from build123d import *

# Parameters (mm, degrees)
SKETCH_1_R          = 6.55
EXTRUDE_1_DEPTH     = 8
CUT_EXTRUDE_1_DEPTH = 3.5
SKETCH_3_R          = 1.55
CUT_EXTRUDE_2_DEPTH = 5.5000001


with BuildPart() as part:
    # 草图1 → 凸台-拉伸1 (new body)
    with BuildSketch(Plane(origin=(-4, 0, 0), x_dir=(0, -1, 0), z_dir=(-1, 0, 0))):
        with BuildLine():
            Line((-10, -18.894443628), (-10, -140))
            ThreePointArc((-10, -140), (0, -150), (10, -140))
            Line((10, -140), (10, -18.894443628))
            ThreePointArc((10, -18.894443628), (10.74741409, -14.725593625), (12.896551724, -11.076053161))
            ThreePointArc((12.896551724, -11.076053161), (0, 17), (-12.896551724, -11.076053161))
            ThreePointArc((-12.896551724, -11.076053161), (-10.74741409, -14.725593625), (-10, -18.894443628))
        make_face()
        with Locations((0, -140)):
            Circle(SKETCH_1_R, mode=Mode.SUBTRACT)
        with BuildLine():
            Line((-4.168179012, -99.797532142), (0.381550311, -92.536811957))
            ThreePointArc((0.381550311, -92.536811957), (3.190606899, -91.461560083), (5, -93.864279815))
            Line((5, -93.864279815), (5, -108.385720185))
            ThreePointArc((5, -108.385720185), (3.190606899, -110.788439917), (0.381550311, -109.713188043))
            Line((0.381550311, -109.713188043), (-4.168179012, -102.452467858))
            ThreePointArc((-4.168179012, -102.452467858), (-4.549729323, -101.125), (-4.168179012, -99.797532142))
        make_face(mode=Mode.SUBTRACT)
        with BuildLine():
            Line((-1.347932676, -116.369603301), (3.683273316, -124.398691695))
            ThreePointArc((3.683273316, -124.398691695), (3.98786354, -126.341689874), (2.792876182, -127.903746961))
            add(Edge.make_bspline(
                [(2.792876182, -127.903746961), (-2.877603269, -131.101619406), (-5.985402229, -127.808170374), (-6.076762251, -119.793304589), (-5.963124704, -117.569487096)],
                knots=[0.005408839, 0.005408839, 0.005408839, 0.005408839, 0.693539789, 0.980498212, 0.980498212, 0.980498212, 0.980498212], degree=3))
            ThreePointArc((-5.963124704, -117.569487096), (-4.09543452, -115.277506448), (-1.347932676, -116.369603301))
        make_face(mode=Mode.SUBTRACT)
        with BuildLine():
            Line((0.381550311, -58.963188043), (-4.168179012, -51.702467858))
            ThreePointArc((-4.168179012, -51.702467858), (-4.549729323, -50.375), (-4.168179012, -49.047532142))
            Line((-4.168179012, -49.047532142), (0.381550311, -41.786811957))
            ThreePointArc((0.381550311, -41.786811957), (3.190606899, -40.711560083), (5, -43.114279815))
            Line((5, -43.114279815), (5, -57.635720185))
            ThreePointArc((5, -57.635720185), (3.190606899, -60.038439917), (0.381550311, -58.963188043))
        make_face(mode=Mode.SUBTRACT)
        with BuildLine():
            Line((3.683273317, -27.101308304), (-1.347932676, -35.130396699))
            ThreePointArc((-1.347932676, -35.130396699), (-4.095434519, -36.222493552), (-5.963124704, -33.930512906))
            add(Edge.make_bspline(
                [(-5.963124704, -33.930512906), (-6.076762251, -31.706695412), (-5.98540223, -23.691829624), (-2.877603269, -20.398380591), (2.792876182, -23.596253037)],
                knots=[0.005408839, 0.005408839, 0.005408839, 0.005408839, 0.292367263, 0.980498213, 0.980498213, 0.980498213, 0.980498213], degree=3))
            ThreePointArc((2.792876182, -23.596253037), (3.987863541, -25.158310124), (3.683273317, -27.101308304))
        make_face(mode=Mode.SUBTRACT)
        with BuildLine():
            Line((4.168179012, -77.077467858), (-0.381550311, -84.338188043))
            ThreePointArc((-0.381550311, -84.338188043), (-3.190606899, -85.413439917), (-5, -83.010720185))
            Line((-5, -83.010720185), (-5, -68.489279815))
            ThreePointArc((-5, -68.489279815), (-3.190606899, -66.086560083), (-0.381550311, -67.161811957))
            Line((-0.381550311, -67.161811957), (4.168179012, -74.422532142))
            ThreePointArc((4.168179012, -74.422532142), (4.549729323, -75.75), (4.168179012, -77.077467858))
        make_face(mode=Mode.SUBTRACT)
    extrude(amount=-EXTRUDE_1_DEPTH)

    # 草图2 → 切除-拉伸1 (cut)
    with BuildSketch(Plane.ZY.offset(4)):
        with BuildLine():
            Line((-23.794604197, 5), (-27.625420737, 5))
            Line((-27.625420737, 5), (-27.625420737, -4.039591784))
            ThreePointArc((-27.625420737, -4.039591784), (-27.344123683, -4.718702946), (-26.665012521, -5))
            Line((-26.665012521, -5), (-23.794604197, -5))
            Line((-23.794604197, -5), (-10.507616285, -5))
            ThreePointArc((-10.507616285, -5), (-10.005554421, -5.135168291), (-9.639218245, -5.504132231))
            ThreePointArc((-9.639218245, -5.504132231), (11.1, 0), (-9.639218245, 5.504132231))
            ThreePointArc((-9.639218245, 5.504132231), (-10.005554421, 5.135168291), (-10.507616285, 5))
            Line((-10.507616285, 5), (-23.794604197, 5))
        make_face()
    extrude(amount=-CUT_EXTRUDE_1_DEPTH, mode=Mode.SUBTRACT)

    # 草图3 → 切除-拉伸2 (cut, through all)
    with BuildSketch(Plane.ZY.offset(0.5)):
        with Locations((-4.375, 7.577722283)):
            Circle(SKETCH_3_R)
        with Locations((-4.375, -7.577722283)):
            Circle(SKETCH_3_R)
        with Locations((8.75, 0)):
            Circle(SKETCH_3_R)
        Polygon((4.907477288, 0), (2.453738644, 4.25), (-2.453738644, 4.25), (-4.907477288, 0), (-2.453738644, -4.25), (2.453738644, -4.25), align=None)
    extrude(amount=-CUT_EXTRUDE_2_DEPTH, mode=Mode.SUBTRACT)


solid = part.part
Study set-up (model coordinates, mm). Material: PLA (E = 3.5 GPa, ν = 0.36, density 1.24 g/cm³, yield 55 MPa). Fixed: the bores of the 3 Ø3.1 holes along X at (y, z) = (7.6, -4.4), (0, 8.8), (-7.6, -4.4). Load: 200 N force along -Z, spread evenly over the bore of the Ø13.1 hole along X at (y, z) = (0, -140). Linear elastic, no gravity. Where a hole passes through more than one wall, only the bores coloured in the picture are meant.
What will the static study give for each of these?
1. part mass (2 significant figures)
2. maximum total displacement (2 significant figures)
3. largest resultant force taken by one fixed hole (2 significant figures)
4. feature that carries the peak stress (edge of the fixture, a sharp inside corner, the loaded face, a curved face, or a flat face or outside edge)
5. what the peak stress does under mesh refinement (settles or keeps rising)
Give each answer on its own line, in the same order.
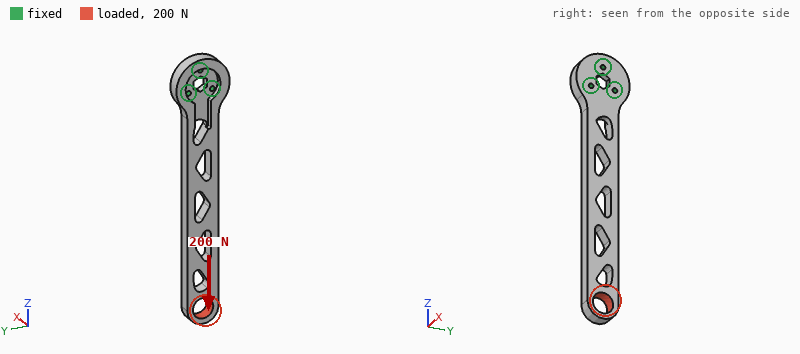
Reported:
25 g
0.29 mm
99 N
edge of the fixture
keeps rising
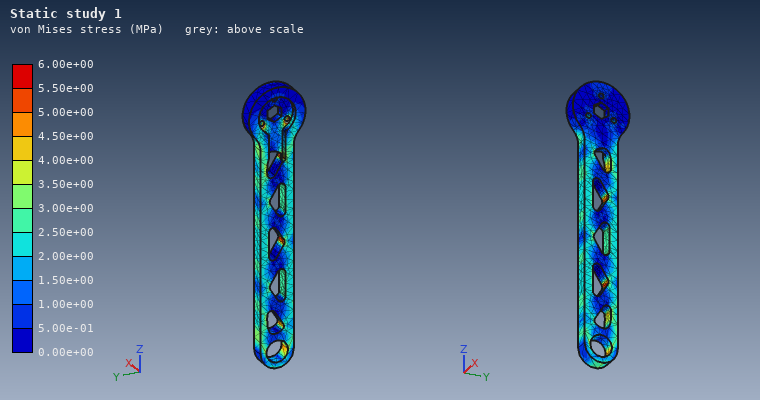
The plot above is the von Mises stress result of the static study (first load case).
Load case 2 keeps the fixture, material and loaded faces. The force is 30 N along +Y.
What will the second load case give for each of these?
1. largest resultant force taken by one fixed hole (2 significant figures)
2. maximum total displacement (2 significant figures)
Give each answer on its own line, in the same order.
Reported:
210 N
1.7 mm
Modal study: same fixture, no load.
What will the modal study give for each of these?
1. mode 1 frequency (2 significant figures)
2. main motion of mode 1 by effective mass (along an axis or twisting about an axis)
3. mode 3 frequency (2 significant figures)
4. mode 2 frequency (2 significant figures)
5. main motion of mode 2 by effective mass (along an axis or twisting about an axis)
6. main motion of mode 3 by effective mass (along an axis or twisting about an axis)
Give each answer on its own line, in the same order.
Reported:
98 Hz
along X
600 Hz
300 Hz
along Y
along X
